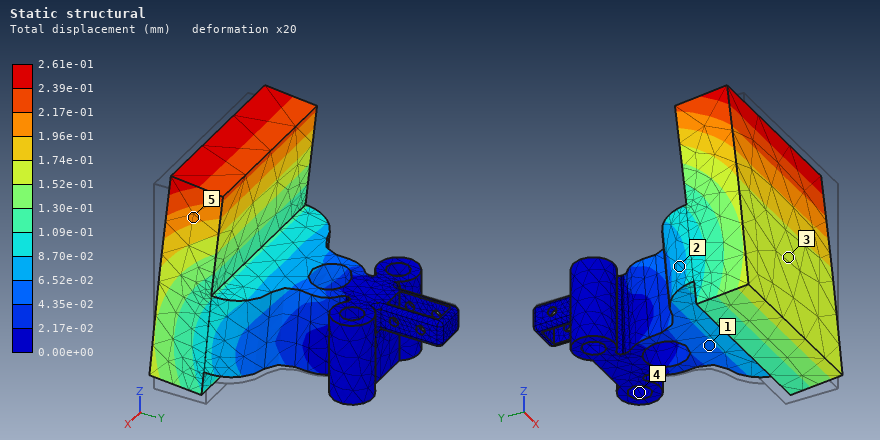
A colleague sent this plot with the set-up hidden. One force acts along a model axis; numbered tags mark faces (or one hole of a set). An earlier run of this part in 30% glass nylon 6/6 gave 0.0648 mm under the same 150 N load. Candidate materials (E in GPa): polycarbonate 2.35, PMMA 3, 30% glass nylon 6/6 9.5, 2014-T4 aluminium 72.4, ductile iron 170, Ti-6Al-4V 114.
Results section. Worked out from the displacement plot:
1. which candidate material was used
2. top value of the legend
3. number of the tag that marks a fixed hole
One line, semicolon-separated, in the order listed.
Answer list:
polycarbonate; 2.61e-01 mm; 4
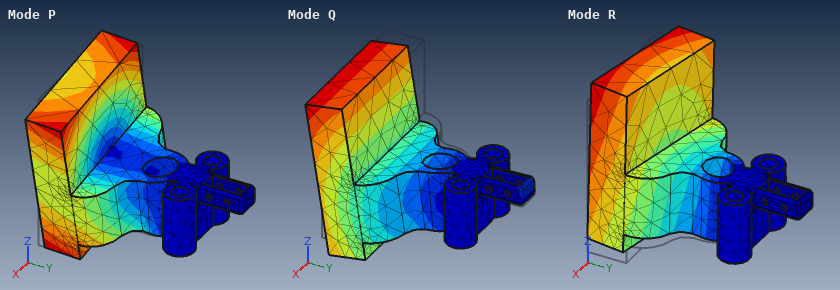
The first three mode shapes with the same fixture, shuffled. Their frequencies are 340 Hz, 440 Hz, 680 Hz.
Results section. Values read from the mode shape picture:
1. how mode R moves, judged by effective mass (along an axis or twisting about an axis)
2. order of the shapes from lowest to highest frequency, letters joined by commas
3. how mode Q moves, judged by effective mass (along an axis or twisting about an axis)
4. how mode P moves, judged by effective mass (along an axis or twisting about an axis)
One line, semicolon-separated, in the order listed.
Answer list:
along X; R, Q, P; along Z; twisting about Y
